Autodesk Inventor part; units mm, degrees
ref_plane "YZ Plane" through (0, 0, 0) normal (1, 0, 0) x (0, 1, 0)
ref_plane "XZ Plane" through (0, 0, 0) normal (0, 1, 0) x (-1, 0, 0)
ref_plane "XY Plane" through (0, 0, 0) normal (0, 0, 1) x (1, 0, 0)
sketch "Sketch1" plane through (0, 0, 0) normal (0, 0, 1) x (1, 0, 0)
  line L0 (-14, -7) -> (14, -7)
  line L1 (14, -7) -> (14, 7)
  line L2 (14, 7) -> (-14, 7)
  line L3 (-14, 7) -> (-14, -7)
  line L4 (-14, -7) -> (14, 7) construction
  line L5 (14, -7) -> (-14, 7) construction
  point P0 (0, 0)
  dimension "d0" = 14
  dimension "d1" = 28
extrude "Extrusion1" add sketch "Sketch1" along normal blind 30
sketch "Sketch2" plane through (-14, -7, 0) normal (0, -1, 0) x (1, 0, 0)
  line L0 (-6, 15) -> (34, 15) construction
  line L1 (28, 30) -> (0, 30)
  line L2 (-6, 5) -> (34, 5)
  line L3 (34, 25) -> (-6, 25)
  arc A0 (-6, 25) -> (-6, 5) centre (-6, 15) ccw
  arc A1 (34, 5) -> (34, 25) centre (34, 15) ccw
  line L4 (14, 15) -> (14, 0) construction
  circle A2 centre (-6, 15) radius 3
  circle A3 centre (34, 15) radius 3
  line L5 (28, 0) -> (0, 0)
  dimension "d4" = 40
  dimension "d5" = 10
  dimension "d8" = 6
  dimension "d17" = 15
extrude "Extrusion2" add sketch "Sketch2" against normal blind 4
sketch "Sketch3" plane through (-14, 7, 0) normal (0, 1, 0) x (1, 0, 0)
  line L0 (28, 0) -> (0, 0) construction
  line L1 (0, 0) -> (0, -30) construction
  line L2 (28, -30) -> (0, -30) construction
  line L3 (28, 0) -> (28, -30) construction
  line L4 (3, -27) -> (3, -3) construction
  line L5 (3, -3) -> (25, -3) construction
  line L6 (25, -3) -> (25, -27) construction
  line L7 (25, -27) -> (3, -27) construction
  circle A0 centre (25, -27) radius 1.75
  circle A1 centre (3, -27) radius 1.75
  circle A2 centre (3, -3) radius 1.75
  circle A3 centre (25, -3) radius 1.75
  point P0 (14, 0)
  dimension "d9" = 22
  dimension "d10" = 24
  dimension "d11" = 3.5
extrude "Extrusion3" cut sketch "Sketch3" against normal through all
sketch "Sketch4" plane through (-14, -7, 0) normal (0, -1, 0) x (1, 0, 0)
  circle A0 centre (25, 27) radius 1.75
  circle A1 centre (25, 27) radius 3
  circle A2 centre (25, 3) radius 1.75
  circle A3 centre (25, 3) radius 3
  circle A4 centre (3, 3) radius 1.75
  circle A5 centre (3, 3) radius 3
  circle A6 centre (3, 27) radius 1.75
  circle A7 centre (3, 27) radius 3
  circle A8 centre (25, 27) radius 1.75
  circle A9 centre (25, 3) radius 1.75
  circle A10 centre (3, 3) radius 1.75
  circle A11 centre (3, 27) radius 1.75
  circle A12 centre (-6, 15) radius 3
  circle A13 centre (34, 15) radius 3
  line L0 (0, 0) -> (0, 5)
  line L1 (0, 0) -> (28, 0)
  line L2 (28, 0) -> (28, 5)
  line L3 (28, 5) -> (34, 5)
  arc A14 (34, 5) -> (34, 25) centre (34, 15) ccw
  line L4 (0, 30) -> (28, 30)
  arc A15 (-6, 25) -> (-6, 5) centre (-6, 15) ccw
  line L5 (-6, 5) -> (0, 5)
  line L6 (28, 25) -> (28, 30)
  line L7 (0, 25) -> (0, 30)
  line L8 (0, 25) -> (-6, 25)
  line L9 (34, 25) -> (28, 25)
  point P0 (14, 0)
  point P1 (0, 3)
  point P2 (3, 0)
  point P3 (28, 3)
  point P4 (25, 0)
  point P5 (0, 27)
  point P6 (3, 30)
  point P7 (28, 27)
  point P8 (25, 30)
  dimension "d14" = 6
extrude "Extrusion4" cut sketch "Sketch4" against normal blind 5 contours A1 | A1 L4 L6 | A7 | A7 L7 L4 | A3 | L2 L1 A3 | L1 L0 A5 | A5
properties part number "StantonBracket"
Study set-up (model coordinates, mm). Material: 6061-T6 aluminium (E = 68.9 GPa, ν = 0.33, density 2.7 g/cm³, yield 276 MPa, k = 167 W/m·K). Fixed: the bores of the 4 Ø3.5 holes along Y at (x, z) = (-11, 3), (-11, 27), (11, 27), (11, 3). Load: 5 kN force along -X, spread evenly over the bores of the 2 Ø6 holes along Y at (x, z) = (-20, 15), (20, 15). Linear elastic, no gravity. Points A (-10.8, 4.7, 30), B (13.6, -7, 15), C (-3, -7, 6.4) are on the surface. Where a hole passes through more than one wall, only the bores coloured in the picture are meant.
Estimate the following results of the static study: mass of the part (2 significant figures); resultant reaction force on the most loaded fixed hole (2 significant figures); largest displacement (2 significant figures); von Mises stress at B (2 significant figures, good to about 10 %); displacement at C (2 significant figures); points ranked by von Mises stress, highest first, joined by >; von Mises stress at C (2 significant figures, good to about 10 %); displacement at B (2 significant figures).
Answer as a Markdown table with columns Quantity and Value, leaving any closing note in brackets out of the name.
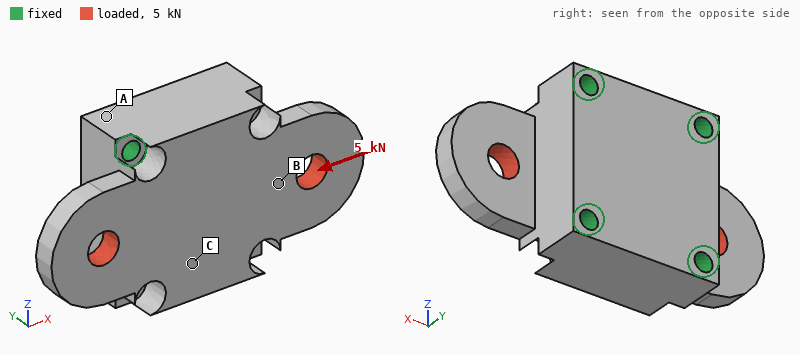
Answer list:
| Quantity | Value |
|---|---|
| mass of the part | 35 g |
| resultant reaction force on the most loaded fixed hole | 1.5 kN |
| largest displacement | 23 µm |
| von Mises stress at B | 38 MPa |
| displacement at C | 3.6 µm |
| points ranked by von Mises stress, highest first, joined by > | B > C > A |
| von Mises stress at C | 16 MPa |
| displacement at B | 9.6 µm |
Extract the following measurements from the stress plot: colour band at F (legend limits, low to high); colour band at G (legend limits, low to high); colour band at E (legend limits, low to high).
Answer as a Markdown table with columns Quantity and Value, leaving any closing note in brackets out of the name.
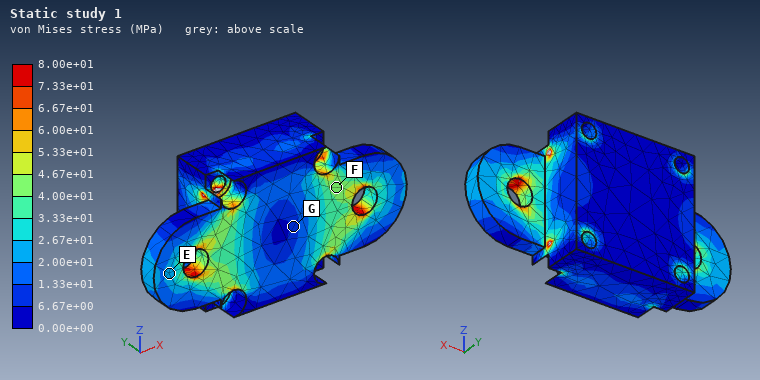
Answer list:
| Quantity | Value |
|---|---|
| colour band at F | 4.00e+01 to 4.67e+01 MPa |
| colour band at G | 6.67e+00 to 1.33e+01 MPa |
| colour band at E | 2.00e+01 to 2.67e+01 MPa |
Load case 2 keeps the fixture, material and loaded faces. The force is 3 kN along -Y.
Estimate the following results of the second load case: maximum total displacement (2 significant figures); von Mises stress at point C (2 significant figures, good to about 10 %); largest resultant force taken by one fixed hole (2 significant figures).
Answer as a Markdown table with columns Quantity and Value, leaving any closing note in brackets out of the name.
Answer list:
| Quantity | Value |
|---|---|
| maximum total displacement | 0.14 mm |
| von Mises stress at point C | 16 MPa |
| largest resultant force taken by one fixed hole | 910 N |
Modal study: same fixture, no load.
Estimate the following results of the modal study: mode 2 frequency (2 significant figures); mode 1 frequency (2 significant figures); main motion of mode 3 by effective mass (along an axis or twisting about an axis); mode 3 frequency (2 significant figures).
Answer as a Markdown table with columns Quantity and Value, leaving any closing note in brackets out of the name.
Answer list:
| Quantity | Value |
|---|---|
| mode 2 frequency | 11 kHz |
| mode 1 frequency | 11 kHz |
| main motion of mode 3 by effective mass | twisting about Y |
| mode 3 frequency | 23 kHz |
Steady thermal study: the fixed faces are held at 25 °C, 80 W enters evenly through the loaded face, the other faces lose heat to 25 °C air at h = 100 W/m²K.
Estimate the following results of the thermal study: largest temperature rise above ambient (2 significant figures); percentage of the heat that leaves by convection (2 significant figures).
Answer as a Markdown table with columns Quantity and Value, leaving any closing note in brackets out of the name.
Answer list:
| Quantity | Value |
|---|---|
| largest temperature rise above ambient | 45 K |
| percentage of the heat that leaves by convection | 7.1 % |
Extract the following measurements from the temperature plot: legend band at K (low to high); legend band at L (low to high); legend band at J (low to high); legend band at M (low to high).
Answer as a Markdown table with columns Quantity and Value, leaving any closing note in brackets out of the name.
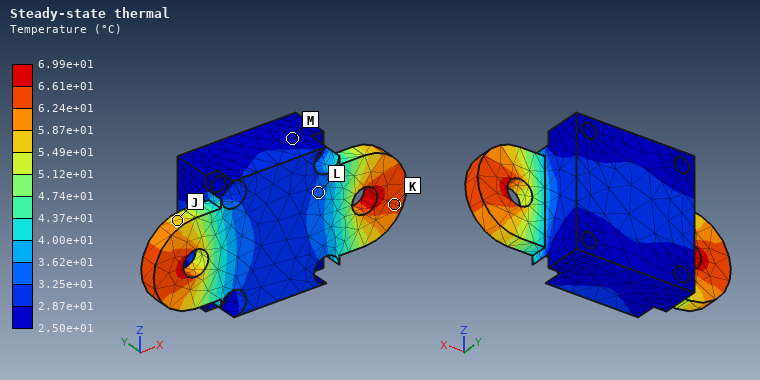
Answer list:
| Quantity | Value |
|---|---|
| legend band at K | 6.24e+01 to 6.61e+01 °C |
| legend band at L | 3.25e+01 to 3.62e+01 °C |
| legend band at J | 5.49e+01 to 5.87e+01 °C |
| legend band at M | 2.50e+01 to 2.87e+01 °C |
